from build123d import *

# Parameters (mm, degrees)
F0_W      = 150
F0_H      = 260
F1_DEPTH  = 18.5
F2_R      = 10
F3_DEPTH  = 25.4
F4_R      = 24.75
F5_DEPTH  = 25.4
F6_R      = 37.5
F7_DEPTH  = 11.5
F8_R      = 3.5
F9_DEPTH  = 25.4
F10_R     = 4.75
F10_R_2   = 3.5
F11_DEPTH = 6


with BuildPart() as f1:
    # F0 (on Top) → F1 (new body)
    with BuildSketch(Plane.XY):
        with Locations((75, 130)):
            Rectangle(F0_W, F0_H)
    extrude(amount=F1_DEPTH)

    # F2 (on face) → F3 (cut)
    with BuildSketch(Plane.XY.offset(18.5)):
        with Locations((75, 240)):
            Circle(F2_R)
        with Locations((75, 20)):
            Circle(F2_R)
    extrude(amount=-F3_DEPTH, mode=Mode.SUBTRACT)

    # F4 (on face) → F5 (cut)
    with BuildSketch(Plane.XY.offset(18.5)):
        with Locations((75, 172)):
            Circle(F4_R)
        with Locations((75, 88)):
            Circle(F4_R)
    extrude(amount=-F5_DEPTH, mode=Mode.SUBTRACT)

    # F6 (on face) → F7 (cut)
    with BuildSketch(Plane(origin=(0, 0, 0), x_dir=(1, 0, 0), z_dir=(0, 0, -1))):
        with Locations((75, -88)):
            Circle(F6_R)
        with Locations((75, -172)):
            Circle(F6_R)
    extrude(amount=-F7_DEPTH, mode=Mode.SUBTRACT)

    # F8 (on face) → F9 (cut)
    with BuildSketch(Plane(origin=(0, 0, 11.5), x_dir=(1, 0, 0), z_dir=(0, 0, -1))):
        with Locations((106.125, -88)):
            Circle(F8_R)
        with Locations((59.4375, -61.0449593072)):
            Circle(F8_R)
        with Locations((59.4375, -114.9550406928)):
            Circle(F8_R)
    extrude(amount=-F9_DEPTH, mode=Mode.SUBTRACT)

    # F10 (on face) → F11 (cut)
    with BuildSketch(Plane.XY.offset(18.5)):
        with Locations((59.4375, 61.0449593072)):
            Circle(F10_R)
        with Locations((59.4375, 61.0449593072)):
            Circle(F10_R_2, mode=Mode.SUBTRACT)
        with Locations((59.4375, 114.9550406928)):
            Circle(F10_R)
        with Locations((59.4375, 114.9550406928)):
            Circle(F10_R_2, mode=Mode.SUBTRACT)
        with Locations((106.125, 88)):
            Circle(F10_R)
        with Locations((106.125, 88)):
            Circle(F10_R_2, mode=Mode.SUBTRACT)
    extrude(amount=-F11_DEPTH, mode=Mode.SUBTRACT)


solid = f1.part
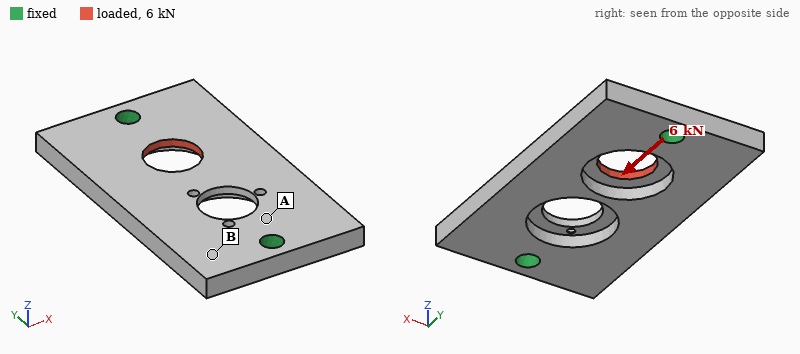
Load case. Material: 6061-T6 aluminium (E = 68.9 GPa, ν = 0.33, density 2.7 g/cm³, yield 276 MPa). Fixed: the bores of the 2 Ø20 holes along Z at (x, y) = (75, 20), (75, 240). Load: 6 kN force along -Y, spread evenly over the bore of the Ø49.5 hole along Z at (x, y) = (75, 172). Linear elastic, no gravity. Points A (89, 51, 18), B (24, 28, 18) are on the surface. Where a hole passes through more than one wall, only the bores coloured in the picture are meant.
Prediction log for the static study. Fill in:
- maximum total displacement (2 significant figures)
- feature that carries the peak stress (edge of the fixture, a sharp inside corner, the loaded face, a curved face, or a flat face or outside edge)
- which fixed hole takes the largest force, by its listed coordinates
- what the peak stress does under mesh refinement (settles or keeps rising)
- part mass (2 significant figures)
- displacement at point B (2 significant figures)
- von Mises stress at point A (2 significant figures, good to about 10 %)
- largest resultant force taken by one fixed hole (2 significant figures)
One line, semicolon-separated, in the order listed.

10 µm; a sharp inside corner; (75, 240); keeps rising; 1.6 kg; 2.7 µm; 2.8 MPa; 4.1 kN
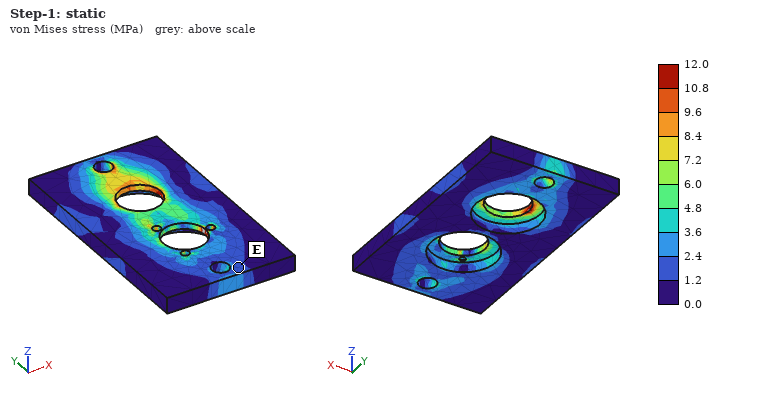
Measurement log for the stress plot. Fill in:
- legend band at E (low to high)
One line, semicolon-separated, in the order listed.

1.2 to 2.4 MPa
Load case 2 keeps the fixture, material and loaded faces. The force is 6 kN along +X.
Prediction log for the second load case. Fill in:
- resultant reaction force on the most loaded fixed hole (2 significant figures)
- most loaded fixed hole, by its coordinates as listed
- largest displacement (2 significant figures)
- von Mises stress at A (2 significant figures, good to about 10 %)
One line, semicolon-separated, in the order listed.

4.2 kN; (75, 240); 16 µm; 4.0 MPa
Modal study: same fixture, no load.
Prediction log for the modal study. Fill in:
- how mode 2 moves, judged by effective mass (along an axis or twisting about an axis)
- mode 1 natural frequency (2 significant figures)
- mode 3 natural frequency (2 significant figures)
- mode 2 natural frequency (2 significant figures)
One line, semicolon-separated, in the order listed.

along Z; 1400 Hz; 2800 Hz; 1500 Hz
